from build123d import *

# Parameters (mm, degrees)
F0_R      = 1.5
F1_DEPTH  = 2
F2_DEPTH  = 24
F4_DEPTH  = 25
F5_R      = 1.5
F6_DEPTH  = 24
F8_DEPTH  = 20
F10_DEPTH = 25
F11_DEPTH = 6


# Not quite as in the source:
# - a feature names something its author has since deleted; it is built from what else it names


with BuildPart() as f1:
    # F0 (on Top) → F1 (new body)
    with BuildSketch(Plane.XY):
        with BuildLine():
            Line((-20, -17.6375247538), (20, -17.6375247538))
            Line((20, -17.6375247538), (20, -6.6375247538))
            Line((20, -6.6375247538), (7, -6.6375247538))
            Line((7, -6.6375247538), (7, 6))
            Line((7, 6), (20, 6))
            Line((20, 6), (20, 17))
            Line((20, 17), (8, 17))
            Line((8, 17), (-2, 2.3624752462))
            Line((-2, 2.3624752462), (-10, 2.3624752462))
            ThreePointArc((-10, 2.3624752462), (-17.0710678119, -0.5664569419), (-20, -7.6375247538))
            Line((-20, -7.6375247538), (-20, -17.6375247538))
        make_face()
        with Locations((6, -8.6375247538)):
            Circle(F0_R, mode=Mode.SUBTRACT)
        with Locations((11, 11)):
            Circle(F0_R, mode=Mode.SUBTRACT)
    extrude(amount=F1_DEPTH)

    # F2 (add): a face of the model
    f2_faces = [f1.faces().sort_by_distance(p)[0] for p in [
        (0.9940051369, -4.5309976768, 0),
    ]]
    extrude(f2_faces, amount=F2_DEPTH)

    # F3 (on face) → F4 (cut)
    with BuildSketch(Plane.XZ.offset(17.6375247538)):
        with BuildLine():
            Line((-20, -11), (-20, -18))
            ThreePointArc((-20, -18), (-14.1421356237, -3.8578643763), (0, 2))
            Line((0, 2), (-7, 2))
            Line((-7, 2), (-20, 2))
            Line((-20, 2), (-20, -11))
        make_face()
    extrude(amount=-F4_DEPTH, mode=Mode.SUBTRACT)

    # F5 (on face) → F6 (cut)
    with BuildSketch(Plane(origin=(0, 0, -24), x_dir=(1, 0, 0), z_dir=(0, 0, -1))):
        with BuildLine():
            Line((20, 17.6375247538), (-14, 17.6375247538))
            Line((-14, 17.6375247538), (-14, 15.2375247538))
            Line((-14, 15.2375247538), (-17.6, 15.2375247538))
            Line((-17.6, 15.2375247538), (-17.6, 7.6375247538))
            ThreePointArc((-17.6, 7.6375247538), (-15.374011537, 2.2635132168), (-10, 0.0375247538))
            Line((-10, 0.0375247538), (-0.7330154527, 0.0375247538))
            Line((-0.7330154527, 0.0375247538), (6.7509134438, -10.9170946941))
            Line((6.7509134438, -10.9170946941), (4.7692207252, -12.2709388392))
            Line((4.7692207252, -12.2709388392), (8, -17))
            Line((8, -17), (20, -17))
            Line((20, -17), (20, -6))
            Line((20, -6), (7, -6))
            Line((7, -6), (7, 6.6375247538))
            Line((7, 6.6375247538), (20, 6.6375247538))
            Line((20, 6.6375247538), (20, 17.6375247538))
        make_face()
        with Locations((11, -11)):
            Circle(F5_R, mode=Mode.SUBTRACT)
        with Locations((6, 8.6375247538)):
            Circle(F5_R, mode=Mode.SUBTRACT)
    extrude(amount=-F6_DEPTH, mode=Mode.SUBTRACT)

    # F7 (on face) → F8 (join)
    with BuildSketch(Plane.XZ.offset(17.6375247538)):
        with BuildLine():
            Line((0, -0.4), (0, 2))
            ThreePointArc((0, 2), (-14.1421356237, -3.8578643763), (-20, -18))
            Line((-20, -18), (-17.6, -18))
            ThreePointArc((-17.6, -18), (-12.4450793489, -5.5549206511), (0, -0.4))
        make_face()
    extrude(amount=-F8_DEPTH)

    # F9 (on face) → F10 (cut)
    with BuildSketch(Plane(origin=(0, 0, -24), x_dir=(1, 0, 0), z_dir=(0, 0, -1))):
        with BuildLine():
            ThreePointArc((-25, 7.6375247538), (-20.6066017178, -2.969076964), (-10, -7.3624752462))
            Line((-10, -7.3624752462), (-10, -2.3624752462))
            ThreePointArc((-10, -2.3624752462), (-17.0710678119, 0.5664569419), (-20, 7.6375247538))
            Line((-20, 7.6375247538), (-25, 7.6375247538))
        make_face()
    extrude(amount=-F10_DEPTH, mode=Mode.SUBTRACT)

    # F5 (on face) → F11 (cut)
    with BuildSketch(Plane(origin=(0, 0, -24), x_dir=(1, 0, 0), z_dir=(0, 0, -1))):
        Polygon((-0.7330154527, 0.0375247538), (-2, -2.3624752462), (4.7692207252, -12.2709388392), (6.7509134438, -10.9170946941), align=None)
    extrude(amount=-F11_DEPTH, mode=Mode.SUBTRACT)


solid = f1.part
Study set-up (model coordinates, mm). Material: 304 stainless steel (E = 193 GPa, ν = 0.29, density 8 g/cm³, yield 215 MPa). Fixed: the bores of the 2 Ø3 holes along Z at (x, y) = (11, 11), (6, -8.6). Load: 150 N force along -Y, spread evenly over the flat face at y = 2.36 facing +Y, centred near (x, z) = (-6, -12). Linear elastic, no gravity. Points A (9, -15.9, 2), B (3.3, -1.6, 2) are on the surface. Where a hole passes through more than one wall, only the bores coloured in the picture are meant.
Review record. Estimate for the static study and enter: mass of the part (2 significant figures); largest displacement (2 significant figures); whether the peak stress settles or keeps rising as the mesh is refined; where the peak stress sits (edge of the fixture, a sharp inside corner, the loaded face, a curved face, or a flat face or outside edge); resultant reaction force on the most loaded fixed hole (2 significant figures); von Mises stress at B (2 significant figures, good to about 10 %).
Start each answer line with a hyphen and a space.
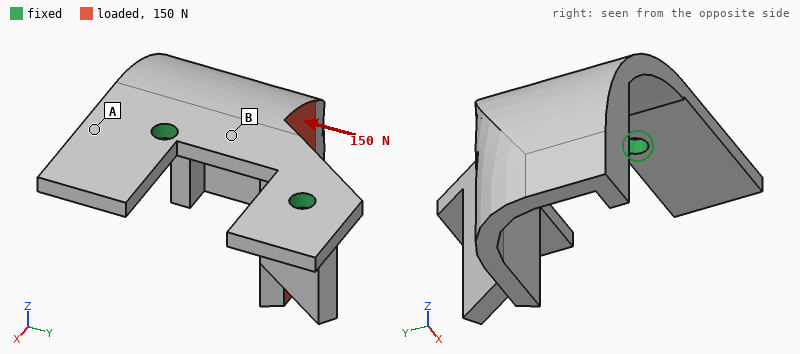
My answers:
- 31 g
- 53 µm
- keeps rising
- edge of the fixture
- 150 N
- 21 MPa
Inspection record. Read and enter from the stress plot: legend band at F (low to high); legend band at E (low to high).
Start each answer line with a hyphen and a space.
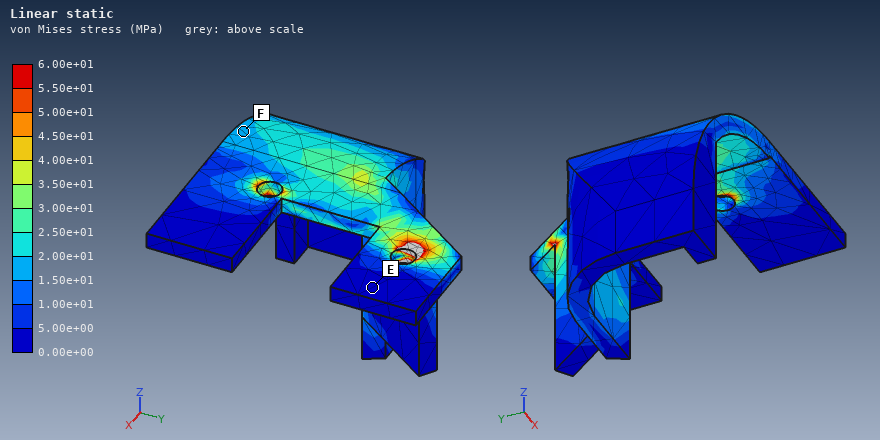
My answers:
- 1.50e+01 to 2.00e+01 MPa
- 0.00e+00 to 5.00e+00 MPa
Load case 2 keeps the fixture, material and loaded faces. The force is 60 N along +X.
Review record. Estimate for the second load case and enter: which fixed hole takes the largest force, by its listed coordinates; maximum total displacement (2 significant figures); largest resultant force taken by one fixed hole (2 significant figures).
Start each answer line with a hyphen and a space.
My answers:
- (11, 11)
- 63 µm
- 44 N
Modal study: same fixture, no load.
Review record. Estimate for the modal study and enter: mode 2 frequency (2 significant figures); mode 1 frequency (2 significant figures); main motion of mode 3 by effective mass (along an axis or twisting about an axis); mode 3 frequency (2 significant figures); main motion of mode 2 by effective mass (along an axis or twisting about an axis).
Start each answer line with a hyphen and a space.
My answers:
- 3100 Hz
- 1100 Hz
- twisting about Z
- 6300 Hz
- along Y
